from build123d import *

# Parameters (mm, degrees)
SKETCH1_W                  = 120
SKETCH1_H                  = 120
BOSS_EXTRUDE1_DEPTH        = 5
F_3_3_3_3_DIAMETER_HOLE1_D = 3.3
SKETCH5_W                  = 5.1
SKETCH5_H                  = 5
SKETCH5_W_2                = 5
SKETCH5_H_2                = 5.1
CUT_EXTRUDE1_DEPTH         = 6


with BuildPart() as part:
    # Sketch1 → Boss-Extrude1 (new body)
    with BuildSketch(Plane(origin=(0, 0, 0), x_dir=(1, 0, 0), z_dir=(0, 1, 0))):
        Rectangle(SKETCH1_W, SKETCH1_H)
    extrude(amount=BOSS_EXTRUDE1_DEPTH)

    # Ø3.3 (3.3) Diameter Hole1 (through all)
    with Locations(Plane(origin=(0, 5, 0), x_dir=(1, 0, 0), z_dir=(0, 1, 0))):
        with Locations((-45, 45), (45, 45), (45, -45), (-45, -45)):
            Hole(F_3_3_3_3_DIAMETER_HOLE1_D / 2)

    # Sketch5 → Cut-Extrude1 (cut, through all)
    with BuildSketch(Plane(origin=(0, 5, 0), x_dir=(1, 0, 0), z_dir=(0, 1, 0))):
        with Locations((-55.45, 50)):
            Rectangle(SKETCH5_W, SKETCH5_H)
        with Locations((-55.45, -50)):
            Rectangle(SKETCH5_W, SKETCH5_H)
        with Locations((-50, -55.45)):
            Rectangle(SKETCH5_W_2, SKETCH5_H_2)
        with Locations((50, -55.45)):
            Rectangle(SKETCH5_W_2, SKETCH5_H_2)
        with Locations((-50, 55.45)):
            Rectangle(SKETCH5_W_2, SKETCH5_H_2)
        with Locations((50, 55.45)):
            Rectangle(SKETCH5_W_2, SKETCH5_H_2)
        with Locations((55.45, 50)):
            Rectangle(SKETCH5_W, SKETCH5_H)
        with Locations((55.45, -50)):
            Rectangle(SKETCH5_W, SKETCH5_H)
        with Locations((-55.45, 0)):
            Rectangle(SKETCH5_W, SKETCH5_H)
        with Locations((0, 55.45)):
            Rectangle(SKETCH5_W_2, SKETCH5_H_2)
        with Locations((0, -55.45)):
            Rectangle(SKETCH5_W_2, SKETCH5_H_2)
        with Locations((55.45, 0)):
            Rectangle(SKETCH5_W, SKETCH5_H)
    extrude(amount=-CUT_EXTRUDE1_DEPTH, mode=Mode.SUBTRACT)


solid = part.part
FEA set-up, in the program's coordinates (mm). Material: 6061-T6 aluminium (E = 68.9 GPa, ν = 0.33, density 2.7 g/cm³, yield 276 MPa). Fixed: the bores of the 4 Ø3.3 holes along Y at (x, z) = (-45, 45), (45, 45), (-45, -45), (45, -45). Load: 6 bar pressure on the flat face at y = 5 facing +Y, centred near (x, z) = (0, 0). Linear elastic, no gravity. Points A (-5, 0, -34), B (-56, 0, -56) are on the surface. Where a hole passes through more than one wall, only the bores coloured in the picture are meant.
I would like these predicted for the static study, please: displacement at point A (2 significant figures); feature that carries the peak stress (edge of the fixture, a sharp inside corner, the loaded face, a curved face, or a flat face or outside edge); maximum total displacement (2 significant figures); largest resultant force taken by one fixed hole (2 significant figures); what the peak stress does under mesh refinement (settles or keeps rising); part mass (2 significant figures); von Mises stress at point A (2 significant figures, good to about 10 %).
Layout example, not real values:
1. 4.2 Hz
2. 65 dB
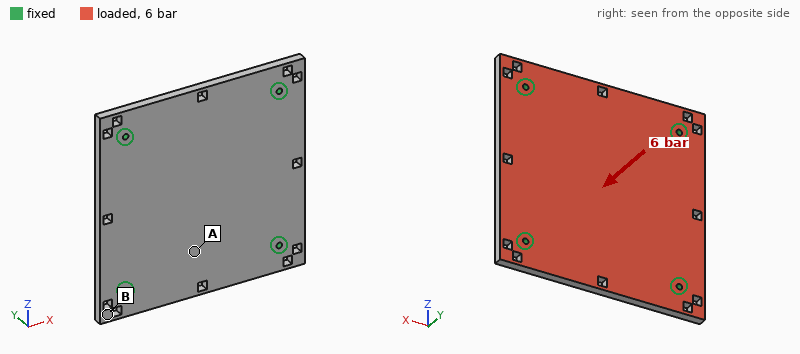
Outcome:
1. 0.30 mm
2. edge of the fixture
3. 0.42 mm
4. 2.1 kN
5. keeps rising
6. 190 g
7. 62 MPa
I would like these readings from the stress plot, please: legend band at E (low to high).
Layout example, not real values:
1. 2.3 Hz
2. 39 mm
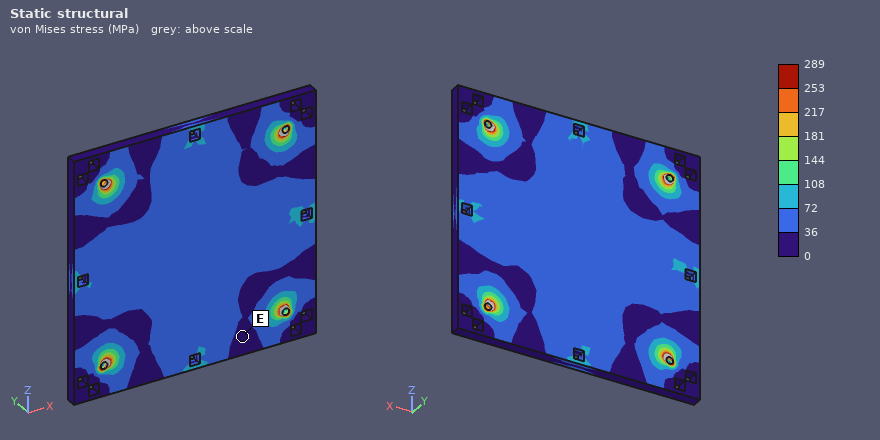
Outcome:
1. 0 to 36 MPa
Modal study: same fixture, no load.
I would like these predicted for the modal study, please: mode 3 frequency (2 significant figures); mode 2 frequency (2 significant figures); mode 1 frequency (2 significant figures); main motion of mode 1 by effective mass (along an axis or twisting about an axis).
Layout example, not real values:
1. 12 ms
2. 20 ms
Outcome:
1. 3100 Hz
2. 3100 Hz
3. 2000 Hz
4. along Y
